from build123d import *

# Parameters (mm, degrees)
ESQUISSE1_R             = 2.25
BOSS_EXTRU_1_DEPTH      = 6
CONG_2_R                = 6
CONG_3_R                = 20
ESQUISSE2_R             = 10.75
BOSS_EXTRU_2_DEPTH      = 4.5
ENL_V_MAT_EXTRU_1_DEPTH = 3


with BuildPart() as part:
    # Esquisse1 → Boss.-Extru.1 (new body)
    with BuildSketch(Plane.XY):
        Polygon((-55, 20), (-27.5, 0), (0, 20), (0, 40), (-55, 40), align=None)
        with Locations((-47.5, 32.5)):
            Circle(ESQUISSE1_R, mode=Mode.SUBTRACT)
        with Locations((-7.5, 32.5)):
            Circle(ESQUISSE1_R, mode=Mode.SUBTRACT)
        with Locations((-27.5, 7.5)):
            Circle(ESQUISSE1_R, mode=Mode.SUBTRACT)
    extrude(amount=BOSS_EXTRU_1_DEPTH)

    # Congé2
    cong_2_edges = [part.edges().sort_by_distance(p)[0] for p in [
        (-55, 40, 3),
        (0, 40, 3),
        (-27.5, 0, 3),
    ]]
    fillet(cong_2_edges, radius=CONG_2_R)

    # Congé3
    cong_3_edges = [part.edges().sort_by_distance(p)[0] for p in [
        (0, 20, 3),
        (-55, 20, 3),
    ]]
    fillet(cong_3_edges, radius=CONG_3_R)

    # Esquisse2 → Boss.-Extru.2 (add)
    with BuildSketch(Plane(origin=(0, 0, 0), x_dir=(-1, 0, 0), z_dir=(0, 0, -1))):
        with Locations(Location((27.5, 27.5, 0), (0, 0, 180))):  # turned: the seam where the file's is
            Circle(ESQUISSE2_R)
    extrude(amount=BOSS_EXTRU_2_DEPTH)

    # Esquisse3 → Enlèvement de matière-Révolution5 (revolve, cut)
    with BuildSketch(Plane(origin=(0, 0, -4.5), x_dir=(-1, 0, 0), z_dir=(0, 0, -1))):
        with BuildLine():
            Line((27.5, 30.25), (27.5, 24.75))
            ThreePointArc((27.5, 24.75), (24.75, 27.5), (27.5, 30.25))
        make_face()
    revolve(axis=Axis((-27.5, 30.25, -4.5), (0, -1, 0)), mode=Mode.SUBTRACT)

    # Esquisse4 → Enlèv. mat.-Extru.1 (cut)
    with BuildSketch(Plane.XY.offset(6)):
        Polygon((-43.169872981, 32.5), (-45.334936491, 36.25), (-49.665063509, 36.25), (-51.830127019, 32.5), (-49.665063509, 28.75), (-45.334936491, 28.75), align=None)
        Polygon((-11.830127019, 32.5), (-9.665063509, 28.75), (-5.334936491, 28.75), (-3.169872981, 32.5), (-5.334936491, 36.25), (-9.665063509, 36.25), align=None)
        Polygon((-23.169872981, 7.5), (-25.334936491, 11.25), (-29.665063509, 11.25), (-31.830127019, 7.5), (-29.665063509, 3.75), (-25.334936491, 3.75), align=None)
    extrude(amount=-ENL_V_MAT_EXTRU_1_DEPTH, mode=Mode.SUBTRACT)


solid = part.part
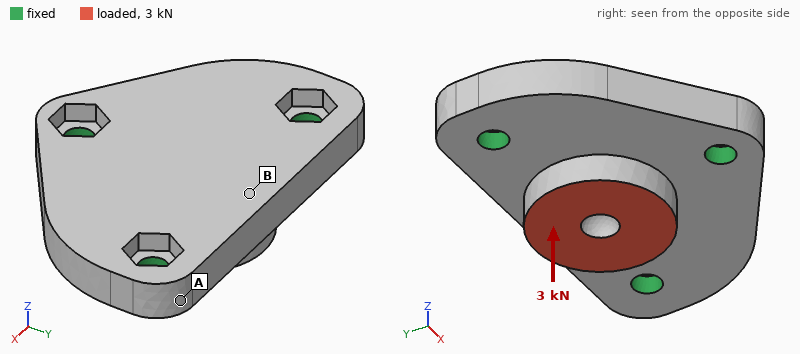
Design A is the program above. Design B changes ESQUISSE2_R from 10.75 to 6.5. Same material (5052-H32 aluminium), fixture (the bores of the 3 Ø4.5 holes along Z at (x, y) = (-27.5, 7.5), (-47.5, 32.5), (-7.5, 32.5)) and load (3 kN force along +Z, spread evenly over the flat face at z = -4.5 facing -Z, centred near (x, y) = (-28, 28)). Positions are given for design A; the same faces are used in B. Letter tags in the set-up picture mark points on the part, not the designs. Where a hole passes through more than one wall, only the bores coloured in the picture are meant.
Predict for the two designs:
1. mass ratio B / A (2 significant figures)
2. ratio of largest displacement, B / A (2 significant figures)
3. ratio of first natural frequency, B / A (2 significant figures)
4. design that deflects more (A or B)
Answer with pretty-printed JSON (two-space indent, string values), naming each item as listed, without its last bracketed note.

{
  "mass ratio B / A": "0.90",
  "ratio of largest displacement, B / A": "1.3",
  "ratio of first natural frequency, B / A": "1.00",
  "design that deflects more": "B"
}
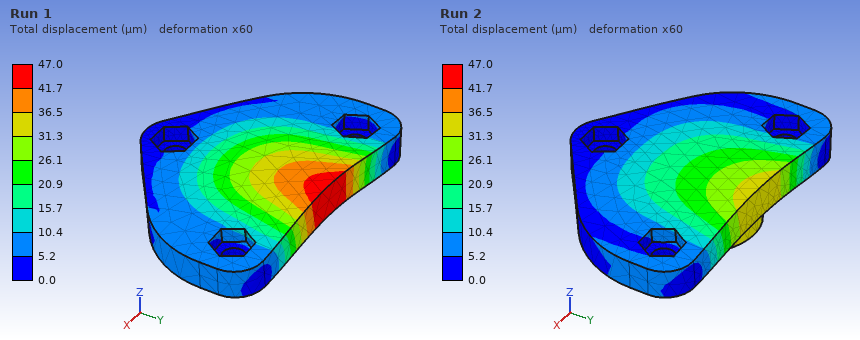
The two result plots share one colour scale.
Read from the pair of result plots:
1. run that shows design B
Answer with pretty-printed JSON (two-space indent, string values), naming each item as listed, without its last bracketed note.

{
  "run that shows design B": "Run 1"
}
